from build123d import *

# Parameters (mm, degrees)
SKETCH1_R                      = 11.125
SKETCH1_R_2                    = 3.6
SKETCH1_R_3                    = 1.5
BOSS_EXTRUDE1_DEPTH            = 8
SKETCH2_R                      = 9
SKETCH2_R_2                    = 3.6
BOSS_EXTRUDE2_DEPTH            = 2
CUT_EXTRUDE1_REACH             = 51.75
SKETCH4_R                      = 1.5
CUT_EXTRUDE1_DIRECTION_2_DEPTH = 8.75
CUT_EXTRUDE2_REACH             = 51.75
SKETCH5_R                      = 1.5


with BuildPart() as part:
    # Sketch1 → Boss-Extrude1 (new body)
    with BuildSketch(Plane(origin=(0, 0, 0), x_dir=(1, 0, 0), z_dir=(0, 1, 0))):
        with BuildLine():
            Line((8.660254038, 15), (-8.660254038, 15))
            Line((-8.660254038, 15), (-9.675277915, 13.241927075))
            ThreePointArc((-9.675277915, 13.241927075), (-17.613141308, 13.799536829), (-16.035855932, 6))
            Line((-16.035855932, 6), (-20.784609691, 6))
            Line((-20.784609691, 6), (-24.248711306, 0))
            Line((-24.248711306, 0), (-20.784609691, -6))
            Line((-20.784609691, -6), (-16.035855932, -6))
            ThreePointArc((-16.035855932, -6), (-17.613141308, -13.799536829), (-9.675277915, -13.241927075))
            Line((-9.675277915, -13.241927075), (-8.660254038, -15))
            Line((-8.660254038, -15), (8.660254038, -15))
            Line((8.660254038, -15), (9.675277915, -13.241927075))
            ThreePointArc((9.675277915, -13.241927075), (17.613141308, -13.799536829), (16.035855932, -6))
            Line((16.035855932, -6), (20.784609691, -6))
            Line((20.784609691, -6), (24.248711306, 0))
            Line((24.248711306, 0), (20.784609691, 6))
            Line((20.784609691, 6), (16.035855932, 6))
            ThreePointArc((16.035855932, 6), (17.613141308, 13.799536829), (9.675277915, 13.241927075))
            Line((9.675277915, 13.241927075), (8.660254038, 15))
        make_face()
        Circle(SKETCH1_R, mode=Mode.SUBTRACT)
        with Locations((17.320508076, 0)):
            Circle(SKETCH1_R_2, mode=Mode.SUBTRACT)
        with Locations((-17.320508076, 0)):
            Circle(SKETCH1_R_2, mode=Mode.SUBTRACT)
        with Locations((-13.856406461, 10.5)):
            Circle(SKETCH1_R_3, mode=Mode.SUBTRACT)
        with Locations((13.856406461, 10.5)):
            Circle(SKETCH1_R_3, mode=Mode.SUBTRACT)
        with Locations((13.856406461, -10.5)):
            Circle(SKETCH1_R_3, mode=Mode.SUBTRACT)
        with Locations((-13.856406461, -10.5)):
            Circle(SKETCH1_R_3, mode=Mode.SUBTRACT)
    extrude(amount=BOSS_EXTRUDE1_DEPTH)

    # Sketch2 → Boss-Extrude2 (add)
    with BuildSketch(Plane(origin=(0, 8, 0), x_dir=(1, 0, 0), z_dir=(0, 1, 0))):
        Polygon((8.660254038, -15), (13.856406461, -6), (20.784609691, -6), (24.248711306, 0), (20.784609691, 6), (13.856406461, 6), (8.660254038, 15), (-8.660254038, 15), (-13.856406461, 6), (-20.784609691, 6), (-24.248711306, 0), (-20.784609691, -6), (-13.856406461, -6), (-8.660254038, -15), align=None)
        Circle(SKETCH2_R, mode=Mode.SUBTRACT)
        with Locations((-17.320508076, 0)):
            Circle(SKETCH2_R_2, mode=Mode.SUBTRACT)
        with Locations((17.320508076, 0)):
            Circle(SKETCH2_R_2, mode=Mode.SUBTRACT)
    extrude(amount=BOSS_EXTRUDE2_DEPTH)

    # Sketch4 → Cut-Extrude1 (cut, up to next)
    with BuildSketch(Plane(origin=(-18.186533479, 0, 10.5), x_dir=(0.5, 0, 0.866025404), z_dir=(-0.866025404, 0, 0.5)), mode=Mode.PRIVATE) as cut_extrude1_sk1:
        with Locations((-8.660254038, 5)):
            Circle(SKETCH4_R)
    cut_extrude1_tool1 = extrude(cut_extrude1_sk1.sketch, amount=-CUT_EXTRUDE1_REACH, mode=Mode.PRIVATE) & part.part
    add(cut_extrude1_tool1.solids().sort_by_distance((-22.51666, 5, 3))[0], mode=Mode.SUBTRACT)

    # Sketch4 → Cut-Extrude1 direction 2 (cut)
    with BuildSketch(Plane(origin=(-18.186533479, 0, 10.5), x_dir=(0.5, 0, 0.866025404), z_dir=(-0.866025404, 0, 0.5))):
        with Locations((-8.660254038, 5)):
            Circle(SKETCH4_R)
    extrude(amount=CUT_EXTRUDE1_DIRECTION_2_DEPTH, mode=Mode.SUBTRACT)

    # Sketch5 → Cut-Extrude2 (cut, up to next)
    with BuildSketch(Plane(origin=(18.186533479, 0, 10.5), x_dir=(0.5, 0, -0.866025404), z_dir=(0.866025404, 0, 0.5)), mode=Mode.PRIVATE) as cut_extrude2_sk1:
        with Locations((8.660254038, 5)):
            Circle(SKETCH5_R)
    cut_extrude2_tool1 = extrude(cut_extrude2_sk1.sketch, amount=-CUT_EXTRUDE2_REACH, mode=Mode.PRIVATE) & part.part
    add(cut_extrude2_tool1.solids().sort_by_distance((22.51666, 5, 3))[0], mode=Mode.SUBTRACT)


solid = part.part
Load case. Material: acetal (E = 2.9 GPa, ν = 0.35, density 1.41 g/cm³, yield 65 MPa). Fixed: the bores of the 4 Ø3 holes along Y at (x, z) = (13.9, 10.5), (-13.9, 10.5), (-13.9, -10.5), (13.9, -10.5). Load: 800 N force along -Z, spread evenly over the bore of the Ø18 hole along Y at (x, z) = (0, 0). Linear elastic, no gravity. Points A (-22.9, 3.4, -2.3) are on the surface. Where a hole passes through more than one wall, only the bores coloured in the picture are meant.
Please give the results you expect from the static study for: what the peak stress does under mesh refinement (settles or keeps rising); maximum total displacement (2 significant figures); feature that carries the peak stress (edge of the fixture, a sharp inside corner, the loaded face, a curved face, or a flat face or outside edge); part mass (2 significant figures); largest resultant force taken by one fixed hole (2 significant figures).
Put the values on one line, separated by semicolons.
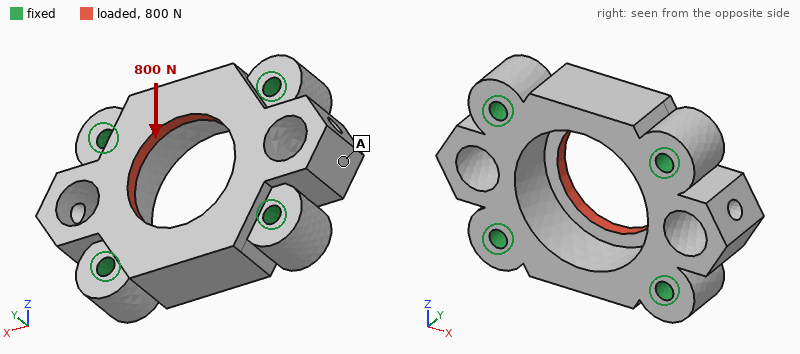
keeps rising; 84 µm; edge of the fixture; 9.4 g; 210 N
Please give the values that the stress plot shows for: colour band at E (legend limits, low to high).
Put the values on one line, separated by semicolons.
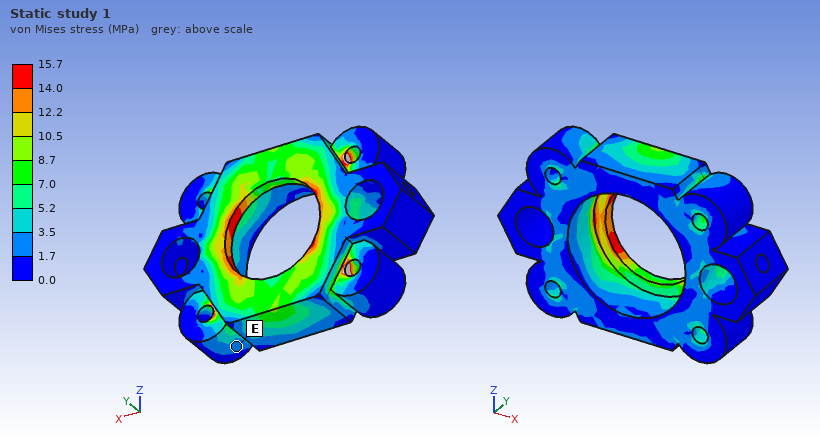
1.7 to 3.5 MPa
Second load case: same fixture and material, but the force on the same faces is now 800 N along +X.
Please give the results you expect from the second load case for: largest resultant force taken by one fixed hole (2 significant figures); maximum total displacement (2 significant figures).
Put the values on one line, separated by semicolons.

210 N; 58 µm
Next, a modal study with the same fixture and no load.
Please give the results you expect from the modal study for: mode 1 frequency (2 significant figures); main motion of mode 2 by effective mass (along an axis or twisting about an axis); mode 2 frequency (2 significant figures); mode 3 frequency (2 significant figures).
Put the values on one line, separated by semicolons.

9100 Hz; twisting about Z; 9700 Hz; 10 kHz
